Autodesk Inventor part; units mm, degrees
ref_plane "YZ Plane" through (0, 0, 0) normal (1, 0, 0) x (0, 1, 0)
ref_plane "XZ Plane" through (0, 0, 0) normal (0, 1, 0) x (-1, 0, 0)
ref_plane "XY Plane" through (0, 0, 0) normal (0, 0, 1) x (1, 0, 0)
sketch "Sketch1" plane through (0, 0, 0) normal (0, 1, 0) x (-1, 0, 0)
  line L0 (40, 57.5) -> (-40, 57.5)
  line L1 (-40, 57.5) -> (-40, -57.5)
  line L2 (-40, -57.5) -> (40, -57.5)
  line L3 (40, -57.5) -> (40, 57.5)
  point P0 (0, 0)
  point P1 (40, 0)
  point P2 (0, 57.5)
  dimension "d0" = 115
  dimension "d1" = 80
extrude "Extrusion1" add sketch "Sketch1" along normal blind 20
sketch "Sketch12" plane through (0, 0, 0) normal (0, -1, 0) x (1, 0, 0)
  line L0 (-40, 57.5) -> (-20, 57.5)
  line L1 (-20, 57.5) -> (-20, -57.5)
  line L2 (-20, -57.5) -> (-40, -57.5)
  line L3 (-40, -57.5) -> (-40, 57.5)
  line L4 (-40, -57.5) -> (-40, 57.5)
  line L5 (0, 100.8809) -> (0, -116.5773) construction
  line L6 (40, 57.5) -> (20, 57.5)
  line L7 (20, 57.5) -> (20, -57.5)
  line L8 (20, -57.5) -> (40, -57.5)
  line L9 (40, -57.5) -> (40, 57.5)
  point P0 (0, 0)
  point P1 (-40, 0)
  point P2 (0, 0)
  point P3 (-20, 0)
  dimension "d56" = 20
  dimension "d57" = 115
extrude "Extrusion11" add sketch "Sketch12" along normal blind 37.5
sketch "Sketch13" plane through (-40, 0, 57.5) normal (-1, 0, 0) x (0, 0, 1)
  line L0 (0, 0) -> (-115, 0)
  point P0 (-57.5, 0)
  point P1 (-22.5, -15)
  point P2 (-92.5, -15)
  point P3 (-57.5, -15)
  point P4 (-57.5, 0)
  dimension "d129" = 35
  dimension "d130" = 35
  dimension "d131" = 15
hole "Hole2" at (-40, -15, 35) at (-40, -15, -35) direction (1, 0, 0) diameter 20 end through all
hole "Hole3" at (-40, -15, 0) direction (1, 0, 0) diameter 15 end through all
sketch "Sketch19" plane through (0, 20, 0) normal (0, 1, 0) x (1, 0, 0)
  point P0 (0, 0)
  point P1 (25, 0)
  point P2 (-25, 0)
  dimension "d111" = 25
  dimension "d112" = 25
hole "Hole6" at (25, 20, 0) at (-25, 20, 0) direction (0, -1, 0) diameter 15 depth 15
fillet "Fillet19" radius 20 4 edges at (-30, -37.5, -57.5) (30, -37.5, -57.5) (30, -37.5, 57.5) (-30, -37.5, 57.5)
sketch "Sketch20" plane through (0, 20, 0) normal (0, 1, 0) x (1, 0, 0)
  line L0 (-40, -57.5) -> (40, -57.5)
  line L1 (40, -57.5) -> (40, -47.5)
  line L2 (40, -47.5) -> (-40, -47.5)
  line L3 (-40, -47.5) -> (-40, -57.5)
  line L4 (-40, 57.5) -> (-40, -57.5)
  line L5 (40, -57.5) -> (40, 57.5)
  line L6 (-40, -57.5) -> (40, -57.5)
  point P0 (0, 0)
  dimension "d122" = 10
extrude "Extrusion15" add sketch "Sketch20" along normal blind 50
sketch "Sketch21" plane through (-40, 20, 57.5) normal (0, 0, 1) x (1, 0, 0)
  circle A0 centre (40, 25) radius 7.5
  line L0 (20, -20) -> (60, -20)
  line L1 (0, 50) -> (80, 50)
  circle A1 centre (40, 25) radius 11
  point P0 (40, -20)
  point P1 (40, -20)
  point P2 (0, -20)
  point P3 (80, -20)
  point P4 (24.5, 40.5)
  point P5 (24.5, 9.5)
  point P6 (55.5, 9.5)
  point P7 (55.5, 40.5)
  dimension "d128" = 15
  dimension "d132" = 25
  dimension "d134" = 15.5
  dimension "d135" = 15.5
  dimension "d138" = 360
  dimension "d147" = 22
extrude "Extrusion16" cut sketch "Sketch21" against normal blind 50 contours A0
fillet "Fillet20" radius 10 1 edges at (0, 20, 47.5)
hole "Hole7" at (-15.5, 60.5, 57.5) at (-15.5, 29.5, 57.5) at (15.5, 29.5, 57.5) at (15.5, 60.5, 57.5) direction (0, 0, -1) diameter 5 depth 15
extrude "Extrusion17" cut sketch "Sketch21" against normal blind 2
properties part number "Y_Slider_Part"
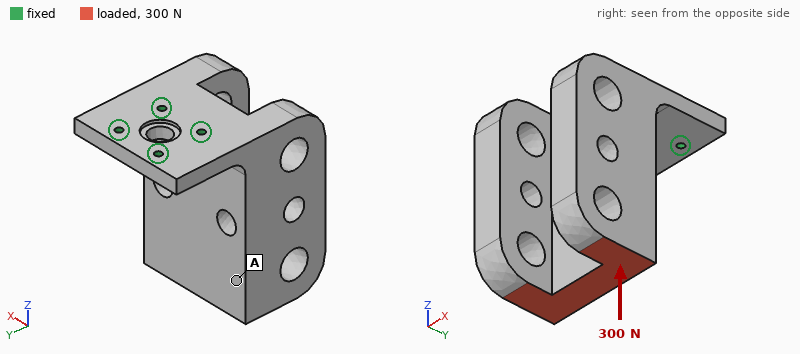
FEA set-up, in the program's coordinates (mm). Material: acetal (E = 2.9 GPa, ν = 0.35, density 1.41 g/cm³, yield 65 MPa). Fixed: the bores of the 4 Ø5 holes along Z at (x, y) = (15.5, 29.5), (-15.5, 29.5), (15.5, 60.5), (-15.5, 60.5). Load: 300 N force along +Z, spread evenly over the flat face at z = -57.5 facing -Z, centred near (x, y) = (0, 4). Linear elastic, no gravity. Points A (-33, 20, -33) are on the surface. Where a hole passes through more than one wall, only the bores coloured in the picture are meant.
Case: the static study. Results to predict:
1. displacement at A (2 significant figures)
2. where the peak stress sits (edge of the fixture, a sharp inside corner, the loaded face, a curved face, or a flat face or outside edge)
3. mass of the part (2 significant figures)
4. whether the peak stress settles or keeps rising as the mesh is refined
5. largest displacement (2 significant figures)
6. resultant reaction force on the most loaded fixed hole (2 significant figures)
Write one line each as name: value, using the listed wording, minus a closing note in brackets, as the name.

displacement at A: 0.33 mm
where the peak stress sits: edge of the fixture
mass of the part: 490 g
whether the peak stress settles or keeps rising as the mesh is refined: keeps rising
largest displacement: 0.47 mm
resultant reaction force on the most loaded fixed hole: 190 N
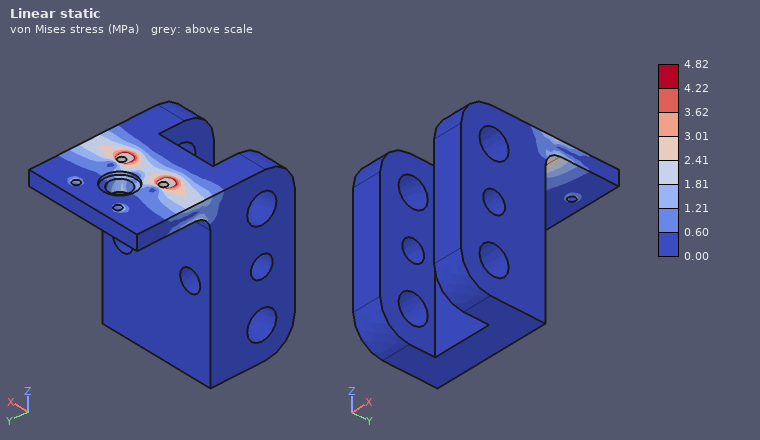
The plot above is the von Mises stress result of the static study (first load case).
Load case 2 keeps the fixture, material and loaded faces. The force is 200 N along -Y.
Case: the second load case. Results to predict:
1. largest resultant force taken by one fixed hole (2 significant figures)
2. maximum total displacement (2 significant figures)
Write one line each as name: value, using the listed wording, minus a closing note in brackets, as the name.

largest resultant force taken by one fixed hole: 170 N
maximum total displacement: 1.7 mm
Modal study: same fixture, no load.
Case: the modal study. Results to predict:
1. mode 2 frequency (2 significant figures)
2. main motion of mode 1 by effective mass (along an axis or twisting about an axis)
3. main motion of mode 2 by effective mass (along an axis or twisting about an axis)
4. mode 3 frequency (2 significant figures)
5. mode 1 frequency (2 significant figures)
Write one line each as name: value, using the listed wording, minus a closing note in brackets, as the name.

mode 2 frequency: 310 Hz
main motion of mode 1 by effective mass: along Y
main motion of mode 2 by effective mass: along X
mode 3 frequency: 570 Hz
mode 1 frequency: 140 Hz
